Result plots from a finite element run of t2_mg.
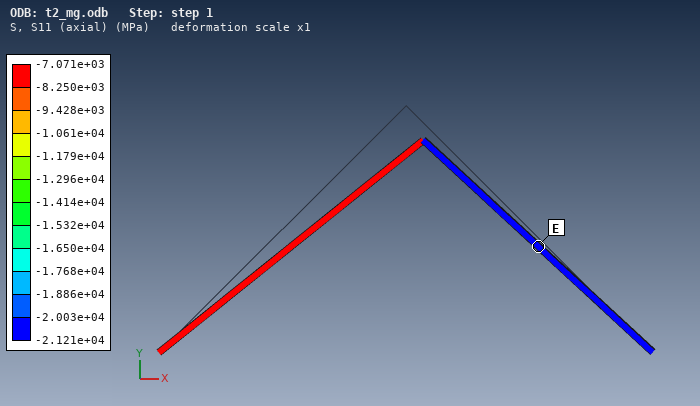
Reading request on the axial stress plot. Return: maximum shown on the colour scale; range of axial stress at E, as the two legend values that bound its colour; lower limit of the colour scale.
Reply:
-7.071e+03 MPa
-2.121e+04 to -2.003e+04 MPa
-2.121e+04 MPa
